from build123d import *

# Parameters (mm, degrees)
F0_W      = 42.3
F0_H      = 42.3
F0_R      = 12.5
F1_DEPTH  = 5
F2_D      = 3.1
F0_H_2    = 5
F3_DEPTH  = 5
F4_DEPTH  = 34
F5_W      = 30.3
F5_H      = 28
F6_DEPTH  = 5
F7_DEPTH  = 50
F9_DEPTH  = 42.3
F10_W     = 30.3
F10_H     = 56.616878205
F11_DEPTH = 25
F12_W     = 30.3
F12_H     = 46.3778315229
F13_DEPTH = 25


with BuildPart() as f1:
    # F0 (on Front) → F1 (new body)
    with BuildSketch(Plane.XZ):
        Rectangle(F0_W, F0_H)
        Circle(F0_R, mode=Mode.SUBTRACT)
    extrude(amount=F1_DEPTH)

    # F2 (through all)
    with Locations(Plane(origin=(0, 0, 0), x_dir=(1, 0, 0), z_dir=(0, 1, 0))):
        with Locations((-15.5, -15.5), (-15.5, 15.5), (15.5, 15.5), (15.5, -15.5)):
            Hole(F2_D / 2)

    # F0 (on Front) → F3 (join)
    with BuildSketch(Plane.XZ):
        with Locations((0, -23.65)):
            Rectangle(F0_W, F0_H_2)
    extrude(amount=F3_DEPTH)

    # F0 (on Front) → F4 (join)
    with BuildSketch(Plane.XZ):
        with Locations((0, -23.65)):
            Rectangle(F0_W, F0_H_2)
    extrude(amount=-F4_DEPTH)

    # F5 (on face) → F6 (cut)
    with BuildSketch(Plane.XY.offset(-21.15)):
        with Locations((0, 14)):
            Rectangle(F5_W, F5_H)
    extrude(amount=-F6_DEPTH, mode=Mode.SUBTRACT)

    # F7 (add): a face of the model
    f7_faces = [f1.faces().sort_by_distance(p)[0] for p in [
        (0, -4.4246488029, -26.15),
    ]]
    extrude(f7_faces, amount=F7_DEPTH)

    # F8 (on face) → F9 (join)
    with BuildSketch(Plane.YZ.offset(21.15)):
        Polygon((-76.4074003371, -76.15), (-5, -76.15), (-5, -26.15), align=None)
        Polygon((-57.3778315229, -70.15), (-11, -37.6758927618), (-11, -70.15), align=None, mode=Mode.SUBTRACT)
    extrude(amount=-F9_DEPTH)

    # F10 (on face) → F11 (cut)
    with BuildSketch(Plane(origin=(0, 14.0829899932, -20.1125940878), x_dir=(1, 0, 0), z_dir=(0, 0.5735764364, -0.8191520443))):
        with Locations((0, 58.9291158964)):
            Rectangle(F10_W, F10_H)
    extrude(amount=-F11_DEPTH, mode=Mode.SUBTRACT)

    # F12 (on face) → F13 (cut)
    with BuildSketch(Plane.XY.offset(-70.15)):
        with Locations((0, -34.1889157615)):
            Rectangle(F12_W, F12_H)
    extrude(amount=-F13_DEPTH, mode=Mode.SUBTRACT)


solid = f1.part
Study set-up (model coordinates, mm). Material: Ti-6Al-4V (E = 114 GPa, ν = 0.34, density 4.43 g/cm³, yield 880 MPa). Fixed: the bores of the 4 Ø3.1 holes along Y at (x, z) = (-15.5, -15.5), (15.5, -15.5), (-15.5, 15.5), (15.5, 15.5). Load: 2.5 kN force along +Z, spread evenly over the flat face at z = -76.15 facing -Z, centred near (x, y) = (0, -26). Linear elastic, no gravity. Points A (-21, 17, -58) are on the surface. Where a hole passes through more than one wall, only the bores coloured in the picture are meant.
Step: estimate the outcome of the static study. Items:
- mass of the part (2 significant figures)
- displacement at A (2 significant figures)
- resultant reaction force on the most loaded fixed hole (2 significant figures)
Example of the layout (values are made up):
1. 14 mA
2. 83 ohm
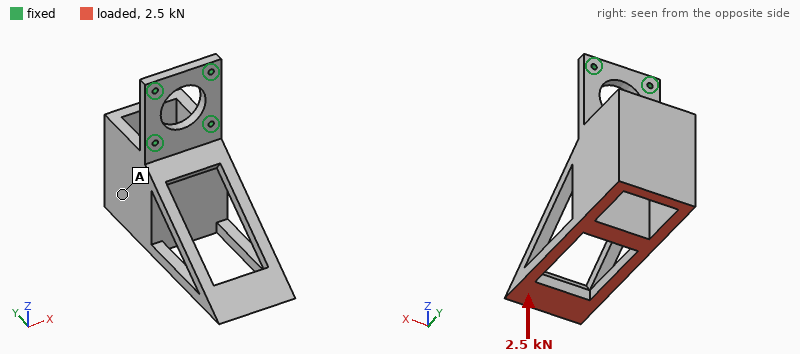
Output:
1. 330 g
2. 0.62 mm
3. 1.3 kN
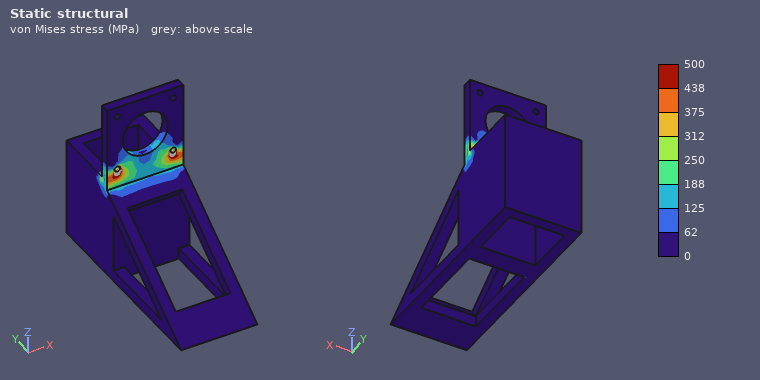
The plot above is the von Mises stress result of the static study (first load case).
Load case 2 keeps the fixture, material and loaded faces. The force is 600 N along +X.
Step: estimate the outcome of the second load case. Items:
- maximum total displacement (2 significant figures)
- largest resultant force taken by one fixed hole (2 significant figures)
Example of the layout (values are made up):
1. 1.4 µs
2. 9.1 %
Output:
1. 0.13 mm
2. 1.2 kN
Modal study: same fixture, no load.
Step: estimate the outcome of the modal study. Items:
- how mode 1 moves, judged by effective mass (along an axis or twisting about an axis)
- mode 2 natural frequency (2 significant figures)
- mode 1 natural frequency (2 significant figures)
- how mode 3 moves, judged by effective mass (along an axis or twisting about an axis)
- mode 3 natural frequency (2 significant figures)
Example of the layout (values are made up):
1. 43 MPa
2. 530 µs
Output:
1. along Y
2. 1300 Hz
3. 410 Hz
4. along X
5. 2200 Hz
